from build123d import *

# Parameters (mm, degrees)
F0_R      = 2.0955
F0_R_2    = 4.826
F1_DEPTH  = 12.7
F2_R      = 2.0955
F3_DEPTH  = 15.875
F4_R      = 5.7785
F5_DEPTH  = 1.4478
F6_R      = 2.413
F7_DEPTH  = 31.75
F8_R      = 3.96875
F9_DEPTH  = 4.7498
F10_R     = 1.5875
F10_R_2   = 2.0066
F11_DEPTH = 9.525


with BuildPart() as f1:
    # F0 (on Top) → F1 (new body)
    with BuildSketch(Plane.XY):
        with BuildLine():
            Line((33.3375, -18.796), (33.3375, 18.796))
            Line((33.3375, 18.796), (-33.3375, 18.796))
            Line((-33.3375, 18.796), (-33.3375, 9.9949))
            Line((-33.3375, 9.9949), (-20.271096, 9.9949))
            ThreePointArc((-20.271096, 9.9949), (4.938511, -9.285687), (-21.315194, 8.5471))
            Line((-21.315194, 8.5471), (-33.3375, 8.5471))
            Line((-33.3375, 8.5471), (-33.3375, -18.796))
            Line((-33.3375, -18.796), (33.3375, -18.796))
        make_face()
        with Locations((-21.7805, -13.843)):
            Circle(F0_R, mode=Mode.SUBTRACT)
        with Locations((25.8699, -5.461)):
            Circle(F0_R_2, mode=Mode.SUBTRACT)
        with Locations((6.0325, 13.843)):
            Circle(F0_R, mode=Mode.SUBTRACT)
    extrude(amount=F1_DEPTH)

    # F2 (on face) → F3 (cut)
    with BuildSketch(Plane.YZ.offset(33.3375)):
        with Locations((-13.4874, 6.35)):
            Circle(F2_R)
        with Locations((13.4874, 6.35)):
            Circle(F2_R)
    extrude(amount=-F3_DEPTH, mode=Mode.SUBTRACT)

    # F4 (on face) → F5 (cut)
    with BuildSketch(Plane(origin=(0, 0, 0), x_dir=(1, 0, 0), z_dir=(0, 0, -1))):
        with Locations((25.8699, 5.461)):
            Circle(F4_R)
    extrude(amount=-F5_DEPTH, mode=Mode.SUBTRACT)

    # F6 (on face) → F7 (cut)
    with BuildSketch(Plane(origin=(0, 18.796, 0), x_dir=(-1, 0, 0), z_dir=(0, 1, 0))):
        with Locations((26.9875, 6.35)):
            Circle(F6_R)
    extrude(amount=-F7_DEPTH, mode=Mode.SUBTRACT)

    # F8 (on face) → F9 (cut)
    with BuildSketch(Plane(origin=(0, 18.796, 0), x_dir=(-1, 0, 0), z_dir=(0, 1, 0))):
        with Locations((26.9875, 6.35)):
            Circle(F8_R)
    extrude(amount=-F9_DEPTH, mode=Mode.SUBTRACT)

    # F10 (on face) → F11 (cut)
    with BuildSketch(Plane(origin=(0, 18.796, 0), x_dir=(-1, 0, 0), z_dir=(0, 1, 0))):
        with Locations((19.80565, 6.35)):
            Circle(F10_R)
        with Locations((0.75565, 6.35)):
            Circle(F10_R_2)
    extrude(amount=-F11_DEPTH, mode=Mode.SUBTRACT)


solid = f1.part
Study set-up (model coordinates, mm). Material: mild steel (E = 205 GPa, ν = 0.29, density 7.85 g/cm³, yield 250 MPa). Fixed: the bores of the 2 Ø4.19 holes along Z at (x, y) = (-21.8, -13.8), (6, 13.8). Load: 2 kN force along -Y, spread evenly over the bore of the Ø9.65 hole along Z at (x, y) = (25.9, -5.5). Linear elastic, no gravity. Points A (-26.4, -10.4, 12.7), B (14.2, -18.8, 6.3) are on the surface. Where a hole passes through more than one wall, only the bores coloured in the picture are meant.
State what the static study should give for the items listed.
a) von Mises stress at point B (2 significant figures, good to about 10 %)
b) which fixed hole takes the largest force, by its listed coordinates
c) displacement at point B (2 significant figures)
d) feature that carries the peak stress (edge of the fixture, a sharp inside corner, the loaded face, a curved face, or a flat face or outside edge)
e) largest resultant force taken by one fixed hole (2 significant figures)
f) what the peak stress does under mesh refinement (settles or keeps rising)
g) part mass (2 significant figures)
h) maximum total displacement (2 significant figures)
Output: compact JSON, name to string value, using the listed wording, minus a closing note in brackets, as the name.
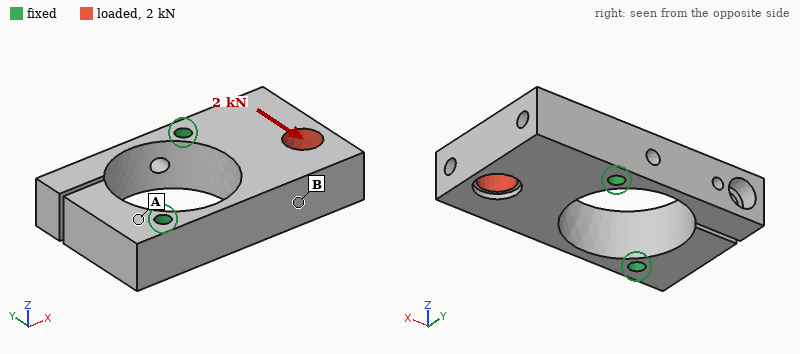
{"von Mises stress at point B": "17 MPa", "which fixed hole takes the largest force, by its listed coordinates": "(6, 13.8)", "displacement at point B": "5.0 µm", "feature that carries the peak stress": "edge of the fixture", "largest resultant force taken by one fixed hole": "2.2 kN", "what the peak stress does under mesh refinement": "keeps rising", "part mass": "150 g", "maximum total displacement": "8.6 µm"}
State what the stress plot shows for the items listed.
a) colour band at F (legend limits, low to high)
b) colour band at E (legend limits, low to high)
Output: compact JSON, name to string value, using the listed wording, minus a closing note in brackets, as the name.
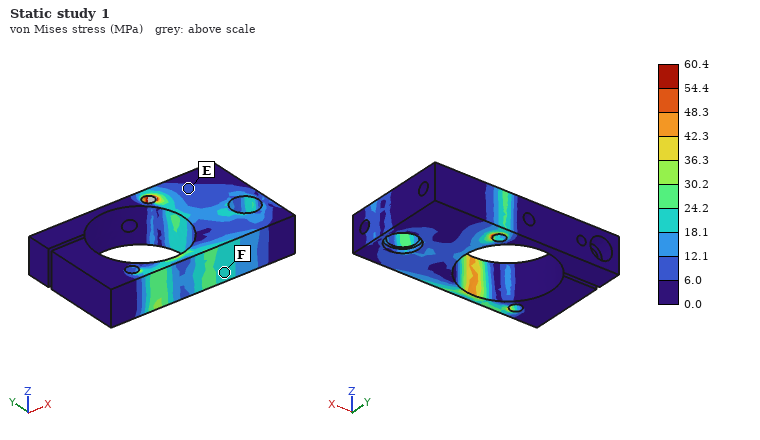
{"colour band at F": "18.1 to 24.2 MPa", "colour band at E": "6.0 to 12.1 MPa"}
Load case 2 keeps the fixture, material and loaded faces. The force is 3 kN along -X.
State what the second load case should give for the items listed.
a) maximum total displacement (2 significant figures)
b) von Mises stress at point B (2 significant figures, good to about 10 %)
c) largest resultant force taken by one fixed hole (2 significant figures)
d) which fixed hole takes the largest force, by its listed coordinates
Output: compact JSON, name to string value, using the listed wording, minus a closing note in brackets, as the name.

{"maximum total displacement": "9.2 µm", "von Mises stress at point B": "23 MPa", "largest resultant force taken by one fixed hole": "1.6 kN", "which fixed hole takes the largest force, by its listed coordinates": "(-21.8, -13.8)"}
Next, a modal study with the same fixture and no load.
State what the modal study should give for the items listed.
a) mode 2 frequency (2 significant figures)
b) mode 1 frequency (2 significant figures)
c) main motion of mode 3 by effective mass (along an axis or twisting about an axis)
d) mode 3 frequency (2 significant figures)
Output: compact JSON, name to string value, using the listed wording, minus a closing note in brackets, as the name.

{"mode 2 frequency": "4500 Hz", "mode 1 frequency": "1600 Hz", "main motion of mode 3 by effective mass": "along Z", "mode 3 frequency": "5900 Hz"}
